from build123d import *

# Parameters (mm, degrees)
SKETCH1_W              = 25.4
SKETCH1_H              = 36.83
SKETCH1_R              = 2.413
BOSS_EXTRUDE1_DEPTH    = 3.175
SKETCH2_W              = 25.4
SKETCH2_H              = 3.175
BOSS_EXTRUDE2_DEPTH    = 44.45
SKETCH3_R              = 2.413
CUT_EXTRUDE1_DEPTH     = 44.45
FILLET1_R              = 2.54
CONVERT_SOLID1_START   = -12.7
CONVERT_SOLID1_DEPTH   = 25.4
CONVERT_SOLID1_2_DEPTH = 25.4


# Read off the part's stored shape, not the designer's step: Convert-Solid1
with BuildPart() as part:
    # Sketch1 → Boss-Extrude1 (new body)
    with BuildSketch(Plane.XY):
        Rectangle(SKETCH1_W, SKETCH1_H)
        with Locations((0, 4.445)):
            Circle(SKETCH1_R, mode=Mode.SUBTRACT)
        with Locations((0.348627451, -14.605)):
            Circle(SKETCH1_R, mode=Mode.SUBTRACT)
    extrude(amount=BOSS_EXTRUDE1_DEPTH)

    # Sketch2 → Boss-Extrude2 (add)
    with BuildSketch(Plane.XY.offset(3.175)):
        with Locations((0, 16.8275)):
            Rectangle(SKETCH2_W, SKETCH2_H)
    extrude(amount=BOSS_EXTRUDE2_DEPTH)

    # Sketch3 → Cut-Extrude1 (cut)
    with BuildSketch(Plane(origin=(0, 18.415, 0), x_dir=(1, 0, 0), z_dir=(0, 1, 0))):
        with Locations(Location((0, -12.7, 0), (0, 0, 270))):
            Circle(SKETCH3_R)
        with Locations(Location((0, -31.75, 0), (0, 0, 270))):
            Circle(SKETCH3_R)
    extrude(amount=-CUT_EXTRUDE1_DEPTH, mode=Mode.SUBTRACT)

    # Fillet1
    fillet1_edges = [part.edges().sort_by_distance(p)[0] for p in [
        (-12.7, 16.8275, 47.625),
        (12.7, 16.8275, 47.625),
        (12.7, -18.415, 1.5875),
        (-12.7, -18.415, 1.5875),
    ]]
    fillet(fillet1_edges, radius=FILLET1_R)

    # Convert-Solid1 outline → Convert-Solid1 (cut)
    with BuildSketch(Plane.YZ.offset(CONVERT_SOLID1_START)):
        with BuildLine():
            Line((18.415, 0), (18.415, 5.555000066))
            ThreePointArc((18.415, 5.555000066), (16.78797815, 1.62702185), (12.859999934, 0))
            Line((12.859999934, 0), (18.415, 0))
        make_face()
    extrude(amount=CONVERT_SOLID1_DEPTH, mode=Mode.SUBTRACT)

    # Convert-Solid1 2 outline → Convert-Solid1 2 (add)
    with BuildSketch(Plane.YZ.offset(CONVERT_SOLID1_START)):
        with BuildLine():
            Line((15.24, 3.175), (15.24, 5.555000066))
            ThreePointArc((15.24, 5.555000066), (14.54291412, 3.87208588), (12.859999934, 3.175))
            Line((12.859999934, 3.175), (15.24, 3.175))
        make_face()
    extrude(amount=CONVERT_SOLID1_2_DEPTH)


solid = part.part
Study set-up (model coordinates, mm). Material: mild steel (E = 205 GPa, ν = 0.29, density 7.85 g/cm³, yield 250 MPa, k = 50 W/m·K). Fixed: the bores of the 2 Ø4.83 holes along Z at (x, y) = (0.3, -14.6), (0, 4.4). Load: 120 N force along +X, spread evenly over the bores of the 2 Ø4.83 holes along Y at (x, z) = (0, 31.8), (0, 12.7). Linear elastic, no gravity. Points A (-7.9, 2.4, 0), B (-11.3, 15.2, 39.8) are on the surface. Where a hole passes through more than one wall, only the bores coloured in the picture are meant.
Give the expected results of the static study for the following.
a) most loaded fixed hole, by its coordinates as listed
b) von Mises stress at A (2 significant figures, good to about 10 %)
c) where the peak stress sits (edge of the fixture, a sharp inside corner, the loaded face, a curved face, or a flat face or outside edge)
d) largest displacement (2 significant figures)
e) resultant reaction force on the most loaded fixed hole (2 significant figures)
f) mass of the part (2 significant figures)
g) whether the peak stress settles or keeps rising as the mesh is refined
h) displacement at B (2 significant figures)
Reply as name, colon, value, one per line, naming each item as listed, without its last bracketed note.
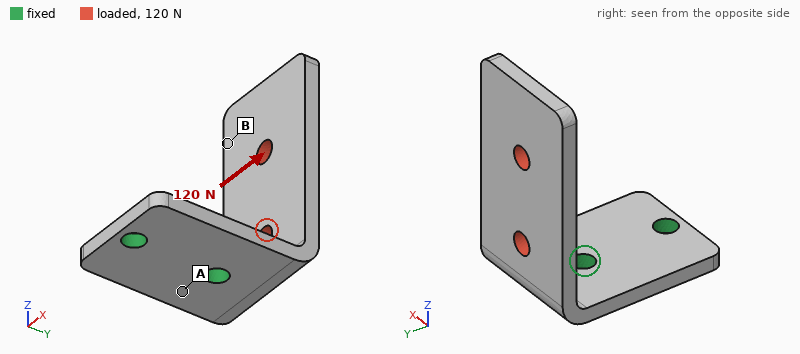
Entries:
most loaded fixed hole, by its coordinates as listed: (0, 4.4)
von Mises stress at A: 27 MPa
where the peak stress sits: edge of the fixture
largest displacement: 54 µm
resultant reaction force on the most loaded fixed hole: 170 N
mass of the part: 48 g
whether the peak stress settles or keeps rising as the mesh is refined: keeps rising
displacement at B: 46 µm
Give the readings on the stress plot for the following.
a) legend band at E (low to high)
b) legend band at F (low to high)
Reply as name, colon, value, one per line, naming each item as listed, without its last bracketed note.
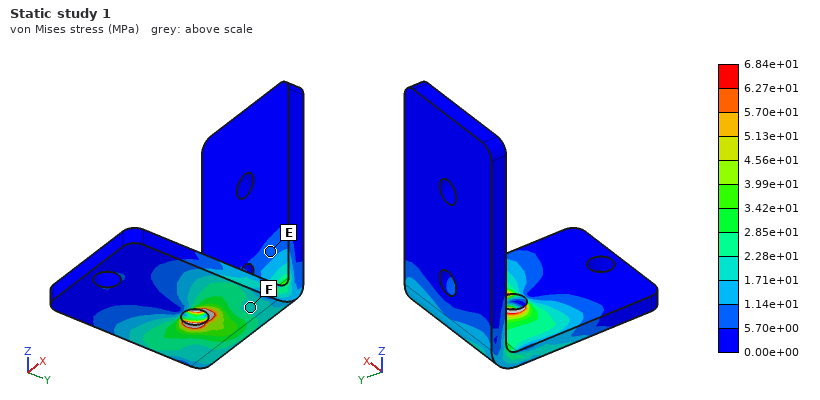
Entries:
legend band at E: 5.70e+00 to 1.14e+01 MPa
legend band at F: 1.71e+01 to 2.28e+01 MPa
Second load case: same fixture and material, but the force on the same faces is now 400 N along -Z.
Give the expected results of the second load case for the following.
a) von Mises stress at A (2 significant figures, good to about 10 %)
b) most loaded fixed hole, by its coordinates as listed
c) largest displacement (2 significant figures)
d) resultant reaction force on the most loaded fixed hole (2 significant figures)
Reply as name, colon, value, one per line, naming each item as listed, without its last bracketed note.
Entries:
von Mises stress at A: 30 MPa
most loaded fixed hole, by its coordinates as listed: (0, 4.4)
largest displacement: 99 µm
resultant reaction force on the most loaded fixed hole: 460 N
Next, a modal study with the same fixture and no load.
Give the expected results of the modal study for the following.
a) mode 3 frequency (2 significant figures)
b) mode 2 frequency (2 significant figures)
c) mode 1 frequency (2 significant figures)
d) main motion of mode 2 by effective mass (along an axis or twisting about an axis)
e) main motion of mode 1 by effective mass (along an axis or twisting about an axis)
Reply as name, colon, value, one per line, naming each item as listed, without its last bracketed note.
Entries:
mode 3 frequency: 4400 Hz
mode 2 frequency: 1600 Hz
mode 1 frequency: 900 Hz
main motion of mode 2 by effective mass: along X
main motion of mode 1 by effective mass: along Y
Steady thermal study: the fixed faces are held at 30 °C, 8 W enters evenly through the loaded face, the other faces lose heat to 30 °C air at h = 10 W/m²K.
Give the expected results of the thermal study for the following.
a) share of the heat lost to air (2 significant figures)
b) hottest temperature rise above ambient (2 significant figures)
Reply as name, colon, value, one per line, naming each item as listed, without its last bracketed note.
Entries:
share of the heat lost to air: 16 %
hottest temperature rise above ambient: 60 K
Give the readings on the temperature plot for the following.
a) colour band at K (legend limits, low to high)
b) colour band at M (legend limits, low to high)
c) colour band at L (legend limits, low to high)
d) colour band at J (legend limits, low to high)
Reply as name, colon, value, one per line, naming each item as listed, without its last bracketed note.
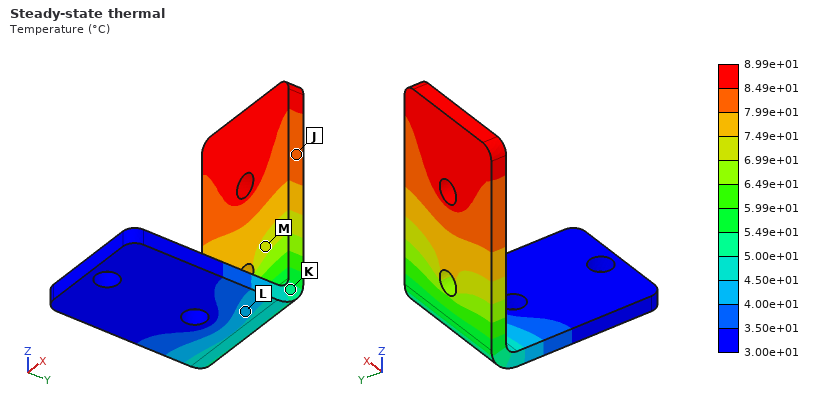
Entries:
colour band at K: 5.00e+01 to 5.49e+01 °C
colour band at M: 6.99e+01 to 7.49e+01 °C
colour band at L: 4.00e+01 to 4.50e+01 °C
colour band at J: 7.99e+01 to 8.49e+01 °C
